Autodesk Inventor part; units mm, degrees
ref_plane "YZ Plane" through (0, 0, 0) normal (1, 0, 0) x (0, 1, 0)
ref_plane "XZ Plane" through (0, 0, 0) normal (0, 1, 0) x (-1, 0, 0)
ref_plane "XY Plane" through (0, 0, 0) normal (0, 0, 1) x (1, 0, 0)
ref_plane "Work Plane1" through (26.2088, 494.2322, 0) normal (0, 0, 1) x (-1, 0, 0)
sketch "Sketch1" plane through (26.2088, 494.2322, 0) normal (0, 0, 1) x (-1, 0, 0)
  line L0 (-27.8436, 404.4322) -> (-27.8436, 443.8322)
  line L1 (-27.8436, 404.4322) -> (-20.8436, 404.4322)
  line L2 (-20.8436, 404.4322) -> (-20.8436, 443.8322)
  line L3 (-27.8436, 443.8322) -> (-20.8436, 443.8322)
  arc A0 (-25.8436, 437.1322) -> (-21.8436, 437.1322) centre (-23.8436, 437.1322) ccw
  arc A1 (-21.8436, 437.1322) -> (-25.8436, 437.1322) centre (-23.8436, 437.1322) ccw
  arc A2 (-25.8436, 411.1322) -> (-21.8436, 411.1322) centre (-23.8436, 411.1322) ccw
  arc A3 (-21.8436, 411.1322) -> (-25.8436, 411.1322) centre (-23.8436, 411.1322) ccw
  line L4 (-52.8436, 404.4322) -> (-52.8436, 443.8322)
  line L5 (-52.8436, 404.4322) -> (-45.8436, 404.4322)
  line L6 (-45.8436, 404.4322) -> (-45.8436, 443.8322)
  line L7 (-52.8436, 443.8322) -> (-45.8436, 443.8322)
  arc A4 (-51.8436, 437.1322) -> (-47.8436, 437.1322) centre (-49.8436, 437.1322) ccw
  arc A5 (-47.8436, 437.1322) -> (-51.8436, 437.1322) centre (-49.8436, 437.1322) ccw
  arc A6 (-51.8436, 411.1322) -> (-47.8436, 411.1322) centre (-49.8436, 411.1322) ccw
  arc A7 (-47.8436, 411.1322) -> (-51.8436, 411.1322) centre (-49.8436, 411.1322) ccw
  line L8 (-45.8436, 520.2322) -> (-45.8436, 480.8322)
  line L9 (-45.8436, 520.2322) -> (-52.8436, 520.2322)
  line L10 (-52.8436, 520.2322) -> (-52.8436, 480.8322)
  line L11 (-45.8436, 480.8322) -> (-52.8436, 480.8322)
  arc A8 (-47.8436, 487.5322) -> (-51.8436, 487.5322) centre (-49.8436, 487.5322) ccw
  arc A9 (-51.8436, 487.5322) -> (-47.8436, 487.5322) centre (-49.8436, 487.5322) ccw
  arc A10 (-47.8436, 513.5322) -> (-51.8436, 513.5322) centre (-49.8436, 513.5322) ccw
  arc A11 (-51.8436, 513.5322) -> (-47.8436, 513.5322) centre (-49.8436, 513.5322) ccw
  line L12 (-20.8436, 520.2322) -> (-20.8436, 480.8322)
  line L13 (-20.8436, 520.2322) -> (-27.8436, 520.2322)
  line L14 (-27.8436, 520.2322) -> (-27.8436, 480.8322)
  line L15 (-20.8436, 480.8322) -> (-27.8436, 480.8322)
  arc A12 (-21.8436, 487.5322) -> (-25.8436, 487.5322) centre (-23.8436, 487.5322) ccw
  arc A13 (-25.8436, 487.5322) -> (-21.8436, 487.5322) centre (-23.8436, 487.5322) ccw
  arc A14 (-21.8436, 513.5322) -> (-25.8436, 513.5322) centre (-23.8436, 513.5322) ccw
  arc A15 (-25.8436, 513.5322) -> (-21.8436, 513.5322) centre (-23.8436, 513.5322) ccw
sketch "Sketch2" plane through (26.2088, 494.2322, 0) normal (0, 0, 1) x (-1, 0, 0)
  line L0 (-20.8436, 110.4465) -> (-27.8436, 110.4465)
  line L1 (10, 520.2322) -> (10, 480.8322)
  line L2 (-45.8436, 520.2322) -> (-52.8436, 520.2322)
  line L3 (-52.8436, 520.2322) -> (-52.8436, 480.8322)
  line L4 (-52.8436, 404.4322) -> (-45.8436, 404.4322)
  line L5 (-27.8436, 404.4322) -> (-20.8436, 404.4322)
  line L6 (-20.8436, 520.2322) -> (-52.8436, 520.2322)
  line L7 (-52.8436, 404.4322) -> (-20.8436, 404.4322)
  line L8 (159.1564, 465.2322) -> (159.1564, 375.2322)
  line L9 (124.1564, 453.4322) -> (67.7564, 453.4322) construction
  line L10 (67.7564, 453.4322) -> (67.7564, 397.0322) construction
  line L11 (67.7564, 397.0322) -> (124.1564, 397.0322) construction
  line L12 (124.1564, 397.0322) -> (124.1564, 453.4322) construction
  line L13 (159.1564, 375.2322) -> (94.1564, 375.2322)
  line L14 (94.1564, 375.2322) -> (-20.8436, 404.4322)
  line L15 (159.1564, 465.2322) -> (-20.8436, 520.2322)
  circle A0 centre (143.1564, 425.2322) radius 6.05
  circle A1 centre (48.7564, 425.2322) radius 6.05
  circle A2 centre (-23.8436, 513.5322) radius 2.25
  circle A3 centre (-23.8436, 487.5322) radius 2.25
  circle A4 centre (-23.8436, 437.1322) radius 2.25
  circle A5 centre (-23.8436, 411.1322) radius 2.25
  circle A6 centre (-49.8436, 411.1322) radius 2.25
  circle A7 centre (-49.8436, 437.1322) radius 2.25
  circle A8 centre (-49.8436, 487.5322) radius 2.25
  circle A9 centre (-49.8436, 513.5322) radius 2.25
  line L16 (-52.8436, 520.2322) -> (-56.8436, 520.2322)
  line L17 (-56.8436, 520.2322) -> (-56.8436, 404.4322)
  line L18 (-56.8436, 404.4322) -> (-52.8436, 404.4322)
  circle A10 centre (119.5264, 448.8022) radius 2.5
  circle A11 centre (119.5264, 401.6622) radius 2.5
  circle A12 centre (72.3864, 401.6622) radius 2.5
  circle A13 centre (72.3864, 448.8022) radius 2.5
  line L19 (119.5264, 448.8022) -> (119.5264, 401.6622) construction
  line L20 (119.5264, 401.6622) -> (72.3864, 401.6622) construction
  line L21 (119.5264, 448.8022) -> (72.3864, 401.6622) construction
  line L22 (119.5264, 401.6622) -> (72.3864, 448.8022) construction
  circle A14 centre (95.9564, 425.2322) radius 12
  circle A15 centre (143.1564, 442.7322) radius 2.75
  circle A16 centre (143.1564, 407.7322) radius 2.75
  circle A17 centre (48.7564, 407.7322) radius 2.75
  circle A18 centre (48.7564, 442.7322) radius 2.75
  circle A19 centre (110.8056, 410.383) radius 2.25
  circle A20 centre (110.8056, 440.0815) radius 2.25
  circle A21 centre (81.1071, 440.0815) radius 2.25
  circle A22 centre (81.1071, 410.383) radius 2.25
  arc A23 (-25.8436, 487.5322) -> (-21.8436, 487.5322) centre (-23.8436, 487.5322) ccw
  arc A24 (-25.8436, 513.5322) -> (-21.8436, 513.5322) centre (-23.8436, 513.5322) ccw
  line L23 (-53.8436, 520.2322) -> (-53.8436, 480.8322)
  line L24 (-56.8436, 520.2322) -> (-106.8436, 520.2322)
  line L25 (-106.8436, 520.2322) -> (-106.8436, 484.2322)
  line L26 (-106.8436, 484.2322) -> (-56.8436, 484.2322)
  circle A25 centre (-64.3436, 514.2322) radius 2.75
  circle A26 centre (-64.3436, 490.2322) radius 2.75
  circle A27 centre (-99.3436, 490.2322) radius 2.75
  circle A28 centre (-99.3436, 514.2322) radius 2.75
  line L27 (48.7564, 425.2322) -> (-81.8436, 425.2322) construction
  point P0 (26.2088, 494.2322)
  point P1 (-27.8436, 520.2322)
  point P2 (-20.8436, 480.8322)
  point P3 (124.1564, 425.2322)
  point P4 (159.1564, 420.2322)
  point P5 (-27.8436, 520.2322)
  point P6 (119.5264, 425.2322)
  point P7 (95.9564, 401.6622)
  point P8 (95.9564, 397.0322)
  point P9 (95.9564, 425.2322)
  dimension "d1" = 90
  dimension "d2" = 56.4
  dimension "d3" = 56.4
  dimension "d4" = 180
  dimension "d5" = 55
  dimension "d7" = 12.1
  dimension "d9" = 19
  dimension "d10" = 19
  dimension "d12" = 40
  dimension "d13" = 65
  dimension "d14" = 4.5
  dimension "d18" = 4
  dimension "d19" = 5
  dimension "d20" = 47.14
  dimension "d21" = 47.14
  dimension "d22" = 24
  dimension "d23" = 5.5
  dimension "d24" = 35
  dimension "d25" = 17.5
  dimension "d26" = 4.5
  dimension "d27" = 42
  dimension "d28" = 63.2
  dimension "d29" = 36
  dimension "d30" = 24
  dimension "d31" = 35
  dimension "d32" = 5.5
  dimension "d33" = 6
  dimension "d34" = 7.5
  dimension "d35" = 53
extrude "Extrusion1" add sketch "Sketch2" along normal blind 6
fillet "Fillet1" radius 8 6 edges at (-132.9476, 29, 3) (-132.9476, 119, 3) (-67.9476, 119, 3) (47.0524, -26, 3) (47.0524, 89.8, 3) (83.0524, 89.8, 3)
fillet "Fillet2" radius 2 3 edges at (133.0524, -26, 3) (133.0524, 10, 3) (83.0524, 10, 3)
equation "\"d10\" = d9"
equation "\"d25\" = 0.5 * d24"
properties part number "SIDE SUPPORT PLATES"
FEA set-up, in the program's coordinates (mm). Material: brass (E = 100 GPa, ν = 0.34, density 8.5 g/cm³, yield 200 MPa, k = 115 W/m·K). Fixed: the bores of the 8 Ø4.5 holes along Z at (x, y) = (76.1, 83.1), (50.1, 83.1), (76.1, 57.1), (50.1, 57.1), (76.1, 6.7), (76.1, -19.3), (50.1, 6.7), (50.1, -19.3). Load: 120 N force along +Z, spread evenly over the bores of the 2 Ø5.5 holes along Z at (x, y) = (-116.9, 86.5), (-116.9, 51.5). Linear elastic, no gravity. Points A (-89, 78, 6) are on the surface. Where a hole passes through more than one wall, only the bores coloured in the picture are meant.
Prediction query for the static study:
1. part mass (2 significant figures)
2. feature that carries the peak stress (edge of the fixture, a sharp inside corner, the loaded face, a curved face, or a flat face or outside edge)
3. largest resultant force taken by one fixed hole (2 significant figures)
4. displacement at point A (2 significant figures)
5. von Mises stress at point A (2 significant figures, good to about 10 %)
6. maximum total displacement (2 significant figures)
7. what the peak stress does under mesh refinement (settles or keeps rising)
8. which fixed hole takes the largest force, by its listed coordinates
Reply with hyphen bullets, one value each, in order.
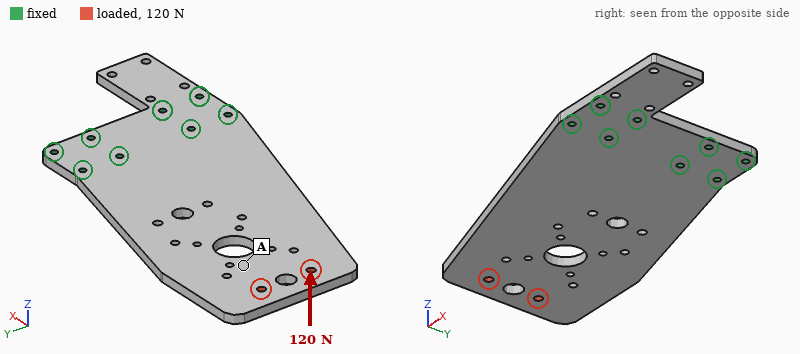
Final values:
- 1.2 kg
- edge of the fixture
- 260 N
- 0.77 mm
- 5.4 MPa
- 1.2 mm
- keeps rising
- (50.1, 57.1)
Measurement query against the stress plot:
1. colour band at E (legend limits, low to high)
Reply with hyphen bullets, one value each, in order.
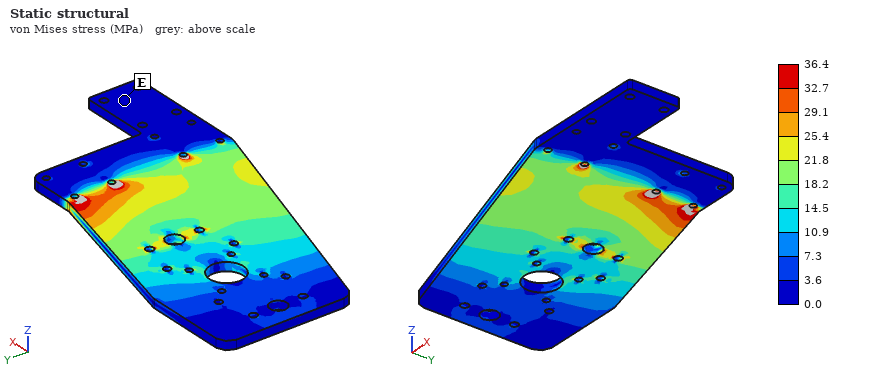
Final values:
- 0.0 to 3.6 MPa
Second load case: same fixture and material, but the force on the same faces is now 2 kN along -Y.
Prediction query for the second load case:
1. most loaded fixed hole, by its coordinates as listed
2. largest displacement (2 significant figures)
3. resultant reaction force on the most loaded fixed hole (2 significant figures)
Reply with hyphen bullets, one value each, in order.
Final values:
- (50.1, 83.1)
- 83 µm
- 2.7 kN
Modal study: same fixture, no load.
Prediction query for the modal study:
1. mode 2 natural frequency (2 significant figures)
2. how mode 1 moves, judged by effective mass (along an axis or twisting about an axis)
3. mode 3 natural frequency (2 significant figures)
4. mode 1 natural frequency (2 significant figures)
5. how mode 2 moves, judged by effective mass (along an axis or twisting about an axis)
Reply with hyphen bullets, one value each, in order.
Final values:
- 390 Hz
- along Z
- 600 Hz
- 110 Hz
- twisting about X
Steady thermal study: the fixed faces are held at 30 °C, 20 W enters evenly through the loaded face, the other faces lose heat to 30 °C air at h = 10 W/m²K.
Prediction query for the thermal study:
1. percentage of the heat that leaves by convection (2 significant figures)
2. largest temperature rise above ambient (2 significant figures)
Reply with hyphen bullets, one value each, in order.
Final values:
- 38 %
- 42 K
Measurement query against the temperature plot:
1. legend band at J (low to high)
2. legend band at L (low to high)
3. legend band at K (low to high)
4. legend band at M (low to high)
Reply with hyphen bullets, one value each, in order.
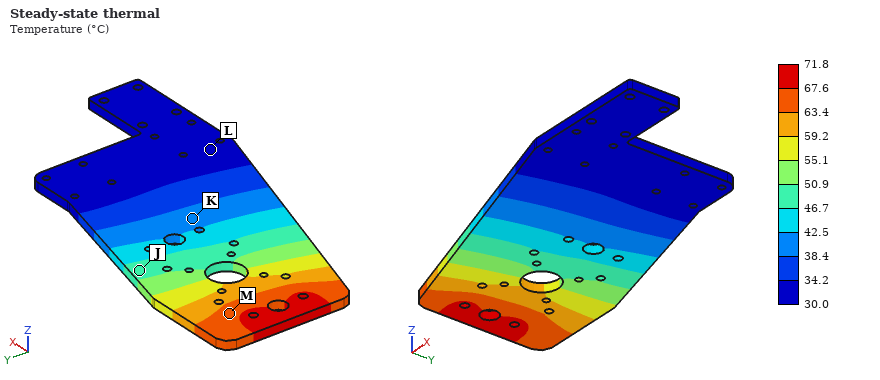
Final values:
- 46.7 to 50.9 °C
- 30.0 to 34.2 °C
- 38.4 to 42.5 °C
- 63.4 to 67.6 °C
